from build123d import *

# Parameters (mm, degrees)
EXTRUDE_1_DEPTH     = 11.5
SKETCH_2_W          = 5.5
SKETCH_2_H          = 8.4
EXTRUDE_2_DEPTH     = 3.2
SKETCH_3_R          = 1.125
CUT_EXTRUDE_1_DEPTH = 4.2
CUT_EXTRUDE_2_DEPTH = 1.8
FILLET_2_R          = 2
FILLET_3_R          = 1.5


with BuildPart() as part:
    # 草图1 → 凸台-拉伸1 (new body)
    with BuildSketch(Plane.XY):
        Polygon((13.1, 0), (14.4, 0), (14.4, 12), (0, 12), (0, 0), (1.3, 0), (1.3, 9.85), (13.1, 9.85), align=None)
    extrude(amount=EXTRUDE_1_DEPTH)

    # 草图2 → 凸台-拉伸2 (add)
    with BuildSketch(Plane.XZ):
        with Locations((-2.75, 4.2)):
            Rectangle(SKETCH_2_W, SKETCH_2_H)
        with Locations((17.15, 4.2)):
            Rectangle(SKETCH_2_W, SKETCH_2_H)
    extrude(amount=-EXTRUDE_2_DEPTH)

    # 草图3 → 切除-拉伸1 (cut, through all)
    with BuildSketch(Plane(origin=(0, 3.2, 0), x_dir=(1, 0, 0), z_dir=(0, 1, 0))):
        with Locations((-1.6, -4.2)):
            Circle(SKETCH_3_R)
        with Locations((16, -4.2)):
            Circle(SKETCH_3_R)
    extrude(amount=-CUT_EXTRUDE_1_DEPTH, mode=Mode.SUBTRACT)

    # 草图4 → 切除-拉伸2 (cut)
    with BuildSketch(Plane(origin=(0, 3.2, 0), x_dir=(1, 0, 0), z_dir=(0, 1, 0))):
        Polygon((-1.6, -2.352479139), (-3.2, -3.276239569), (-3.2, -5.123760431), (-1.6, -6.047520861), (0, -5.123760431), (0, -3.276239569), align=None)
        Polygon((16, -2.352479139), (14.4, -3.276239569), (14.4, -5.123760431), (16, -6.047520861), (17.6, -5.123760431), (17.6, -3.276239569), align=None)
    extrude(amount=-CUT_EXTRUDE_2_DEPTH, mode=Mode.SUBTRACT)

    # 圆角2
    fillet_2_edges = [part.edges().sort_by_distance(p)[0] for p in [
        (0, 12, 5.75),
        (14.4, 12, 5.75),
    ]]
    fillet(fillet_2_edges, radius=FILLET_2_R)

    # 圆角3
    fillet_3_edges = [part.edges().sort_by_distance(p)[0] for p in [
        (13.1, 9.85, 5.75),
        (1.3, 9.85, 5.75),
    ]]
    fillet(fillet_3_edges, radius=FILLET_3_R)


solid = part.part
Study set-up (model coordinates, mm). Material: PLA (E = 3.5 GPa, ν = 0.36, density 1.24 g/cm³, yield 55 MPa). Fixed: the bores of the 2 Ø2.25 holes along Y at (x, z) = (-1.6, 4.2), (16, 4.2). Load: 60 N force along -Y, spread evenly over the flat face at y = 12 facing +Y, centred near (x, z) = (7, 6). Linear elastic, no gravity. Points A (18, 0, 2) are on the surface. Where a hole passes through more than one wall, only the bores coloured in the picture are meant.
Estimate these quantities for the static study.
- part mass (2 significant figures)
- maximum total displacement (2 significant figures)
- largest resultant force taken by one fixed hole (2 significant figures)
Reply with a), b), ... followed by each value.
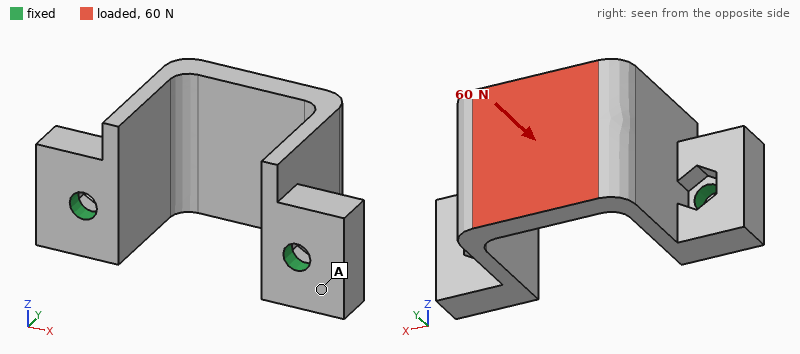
a) 1.1 g
b) 83 µm
c) 31 N
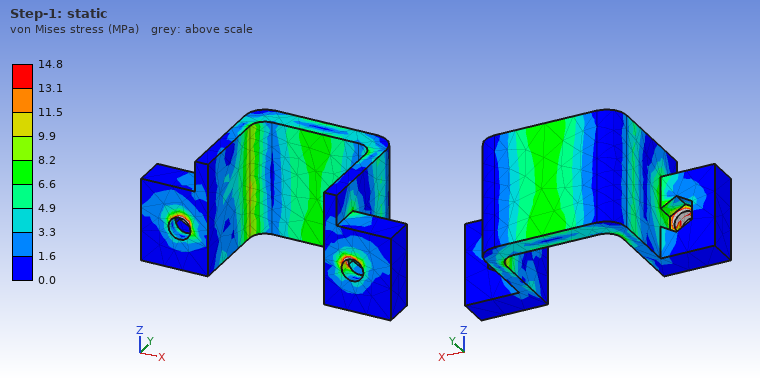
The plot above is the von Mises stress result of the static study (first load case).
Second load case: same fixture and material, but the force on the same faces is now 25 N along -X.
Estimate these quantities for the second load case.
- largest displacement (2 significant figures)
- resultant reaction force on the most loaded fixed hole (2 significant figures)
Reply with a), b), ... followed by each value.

a) 87 µm
b) 17 N
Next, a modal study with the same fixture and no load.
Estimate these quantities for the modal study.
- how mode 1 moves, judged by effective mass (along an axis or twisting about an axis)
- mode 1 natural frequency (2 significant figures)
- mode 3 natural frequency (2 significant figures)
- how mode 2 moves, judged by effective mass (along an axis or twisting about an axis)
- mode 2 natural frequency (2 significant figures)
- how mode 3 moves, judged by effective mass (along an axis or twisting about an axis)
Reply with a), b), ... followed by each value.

a) along Z
b) 3100 Hz
c) 5500 Hz
d) along X
e) 3700 Hz
f) twisting about Y
